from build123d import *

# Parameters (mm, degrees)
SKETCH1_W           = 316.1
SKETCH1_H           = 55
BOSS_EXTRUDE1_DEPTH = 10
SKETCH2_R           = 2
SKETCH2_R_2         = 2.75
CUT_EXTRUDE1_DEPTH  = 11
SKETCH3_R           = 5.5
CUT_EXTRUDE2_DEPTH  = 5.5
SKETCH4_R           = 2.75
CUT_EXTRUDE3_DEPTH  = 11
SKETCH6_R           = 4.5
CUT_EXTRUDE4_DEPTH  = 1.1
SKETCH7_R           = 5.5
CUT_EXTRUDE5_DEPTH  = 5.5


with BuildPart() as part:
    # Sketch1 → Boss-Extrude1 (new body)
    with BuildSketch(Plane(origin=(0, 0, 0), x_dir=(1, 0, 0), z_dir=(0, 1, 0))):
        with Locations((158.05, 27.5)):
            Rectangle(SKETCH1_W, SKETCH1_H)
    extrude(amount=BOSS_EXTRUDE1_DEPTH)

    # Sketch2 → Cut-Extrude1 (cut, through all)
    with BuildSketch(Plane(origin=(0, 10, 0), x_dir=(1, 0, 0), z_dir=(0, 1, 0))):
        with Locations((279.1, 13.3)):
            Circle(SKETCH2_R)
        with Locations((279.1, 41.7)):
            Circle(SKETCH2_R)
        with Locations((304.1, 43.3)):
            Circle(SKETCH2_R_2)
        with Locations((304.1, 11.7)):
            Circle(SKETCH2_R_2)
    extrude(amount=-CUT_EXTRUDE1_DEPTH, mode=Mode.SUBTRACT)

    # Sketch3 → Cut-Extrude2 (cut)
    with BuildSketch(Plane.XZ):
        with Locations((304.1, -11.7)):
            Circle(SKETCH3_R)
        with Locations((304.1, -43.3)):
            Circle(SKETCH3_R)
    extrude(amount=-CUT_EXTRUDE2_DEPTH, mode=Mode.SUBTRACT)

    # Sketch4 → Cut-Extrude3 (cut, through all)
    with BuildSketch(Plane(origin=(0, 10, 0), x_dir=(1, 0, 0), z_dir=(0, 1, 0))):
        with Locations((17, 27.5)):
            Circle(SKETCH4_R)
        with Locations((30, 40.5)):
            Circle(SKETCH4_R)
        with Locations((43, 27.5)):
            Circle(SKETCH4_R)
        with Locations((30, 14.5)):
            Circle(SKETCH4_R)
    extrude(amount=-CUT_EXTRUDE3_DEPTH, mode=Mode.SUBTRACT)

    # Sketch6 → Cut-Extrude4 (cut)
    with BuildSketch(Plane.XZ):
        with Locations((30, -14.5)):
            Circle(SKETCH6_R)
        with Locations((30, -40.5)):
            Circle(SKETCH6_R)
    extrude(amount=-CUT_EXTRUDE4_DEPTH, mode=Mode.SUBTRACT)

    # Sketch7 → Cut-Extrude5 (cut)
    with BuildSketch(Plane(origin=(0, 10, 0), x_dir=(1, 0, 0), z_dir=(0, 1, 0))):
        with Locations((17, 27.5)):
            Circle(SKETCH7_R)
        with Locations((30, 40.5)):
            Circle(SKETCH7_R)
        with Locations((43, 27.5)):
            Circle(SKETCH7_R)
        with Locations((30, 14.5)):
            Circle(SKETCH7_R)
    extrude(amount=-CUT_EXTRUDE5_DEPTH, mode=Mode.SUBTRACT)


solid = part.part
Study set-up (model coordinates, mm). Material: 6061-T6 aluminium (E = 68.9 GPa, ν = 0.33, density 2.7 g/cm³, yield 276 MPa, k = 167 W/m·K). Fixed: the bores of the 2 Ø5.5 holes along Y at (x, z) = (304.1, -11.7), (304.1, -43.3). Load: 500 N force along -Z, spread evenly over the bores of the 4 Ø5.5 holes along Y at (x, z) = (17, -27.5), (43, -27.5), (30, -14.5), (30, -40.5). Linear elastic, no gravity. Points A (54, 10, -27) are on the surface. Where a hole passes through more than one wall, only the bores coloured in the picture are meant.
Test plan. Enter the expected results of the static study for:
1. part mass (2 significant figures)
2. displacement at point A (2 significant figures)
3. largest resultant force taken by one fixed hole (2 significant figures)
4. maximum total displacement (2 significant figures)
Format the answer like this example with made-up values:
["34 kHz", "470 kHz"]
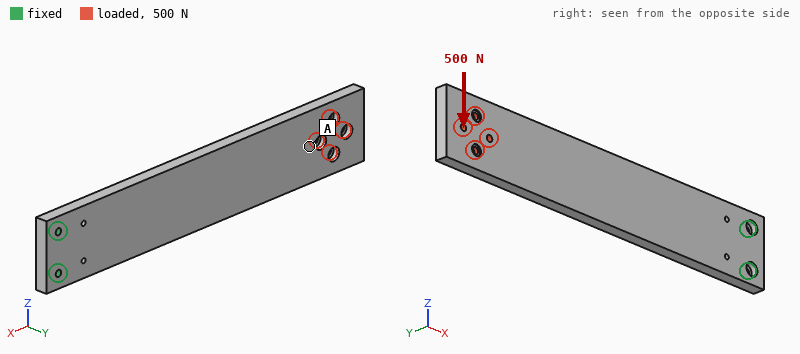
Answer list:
["460 g", "0.40 mm", "4.0 kN", "0.53 mm"]
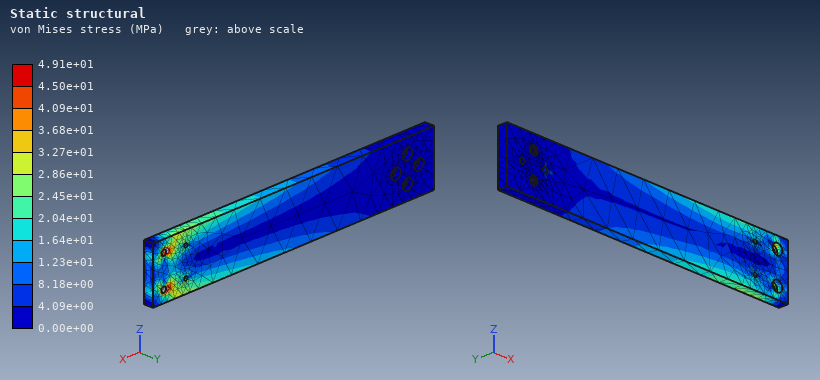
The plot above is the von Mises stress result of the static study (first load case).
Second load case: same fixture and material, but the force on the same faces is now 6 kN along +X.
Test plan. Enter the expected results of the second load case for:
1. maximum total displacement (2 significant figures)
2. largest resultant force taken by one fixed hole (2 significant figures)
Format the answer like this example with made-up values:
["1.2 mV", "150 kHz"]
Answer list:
["3.0 mm", "3.0 kN"]
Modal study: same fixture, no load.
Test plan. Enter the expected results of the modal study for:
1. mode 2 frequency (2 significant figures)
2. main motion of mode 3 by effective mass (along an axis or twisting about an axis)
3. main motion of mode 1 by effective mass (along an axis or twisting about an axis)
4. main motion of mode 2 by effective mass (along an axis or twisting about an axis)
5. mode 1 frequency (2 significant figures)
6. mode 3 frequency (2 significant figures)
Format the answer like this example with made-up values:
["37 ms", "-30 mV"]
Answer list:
["430 Hz", "along Y", "along Y", "along Z", "79 Hz", "500 Hz"]
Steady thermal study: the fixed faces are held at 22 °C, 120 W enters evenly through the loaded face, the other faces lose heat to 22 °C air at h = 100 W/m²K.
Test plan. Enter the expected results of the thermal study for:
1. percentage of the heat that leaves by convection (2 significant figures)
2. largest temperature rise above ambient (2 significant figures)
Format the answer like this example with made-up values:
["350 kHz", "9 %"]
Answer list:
["95 %", "84 K"]
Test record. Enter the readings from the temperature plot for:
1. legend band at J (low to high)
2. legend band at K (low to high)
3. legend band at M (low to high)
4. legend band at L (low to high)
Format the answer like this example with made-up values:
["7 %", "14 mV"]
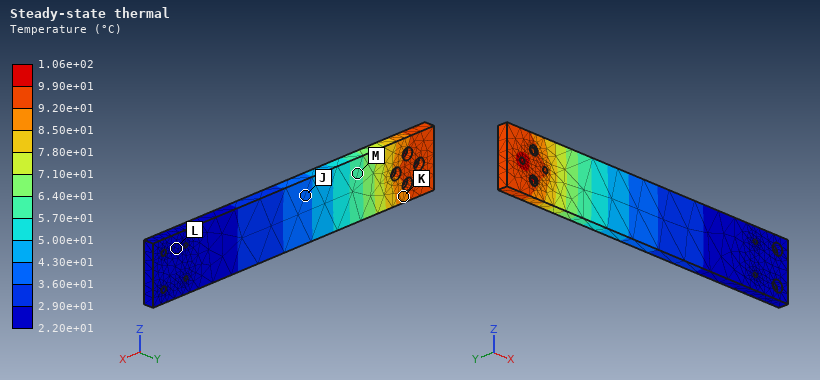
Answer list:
["3.60e+01 to 4.30e+01 °C", "8.50e+01 to 9.20e+01 °C", "5.70e+01 to 6.40e+01 °C", "2.20e+01 to 2.90e+01 °C"]
